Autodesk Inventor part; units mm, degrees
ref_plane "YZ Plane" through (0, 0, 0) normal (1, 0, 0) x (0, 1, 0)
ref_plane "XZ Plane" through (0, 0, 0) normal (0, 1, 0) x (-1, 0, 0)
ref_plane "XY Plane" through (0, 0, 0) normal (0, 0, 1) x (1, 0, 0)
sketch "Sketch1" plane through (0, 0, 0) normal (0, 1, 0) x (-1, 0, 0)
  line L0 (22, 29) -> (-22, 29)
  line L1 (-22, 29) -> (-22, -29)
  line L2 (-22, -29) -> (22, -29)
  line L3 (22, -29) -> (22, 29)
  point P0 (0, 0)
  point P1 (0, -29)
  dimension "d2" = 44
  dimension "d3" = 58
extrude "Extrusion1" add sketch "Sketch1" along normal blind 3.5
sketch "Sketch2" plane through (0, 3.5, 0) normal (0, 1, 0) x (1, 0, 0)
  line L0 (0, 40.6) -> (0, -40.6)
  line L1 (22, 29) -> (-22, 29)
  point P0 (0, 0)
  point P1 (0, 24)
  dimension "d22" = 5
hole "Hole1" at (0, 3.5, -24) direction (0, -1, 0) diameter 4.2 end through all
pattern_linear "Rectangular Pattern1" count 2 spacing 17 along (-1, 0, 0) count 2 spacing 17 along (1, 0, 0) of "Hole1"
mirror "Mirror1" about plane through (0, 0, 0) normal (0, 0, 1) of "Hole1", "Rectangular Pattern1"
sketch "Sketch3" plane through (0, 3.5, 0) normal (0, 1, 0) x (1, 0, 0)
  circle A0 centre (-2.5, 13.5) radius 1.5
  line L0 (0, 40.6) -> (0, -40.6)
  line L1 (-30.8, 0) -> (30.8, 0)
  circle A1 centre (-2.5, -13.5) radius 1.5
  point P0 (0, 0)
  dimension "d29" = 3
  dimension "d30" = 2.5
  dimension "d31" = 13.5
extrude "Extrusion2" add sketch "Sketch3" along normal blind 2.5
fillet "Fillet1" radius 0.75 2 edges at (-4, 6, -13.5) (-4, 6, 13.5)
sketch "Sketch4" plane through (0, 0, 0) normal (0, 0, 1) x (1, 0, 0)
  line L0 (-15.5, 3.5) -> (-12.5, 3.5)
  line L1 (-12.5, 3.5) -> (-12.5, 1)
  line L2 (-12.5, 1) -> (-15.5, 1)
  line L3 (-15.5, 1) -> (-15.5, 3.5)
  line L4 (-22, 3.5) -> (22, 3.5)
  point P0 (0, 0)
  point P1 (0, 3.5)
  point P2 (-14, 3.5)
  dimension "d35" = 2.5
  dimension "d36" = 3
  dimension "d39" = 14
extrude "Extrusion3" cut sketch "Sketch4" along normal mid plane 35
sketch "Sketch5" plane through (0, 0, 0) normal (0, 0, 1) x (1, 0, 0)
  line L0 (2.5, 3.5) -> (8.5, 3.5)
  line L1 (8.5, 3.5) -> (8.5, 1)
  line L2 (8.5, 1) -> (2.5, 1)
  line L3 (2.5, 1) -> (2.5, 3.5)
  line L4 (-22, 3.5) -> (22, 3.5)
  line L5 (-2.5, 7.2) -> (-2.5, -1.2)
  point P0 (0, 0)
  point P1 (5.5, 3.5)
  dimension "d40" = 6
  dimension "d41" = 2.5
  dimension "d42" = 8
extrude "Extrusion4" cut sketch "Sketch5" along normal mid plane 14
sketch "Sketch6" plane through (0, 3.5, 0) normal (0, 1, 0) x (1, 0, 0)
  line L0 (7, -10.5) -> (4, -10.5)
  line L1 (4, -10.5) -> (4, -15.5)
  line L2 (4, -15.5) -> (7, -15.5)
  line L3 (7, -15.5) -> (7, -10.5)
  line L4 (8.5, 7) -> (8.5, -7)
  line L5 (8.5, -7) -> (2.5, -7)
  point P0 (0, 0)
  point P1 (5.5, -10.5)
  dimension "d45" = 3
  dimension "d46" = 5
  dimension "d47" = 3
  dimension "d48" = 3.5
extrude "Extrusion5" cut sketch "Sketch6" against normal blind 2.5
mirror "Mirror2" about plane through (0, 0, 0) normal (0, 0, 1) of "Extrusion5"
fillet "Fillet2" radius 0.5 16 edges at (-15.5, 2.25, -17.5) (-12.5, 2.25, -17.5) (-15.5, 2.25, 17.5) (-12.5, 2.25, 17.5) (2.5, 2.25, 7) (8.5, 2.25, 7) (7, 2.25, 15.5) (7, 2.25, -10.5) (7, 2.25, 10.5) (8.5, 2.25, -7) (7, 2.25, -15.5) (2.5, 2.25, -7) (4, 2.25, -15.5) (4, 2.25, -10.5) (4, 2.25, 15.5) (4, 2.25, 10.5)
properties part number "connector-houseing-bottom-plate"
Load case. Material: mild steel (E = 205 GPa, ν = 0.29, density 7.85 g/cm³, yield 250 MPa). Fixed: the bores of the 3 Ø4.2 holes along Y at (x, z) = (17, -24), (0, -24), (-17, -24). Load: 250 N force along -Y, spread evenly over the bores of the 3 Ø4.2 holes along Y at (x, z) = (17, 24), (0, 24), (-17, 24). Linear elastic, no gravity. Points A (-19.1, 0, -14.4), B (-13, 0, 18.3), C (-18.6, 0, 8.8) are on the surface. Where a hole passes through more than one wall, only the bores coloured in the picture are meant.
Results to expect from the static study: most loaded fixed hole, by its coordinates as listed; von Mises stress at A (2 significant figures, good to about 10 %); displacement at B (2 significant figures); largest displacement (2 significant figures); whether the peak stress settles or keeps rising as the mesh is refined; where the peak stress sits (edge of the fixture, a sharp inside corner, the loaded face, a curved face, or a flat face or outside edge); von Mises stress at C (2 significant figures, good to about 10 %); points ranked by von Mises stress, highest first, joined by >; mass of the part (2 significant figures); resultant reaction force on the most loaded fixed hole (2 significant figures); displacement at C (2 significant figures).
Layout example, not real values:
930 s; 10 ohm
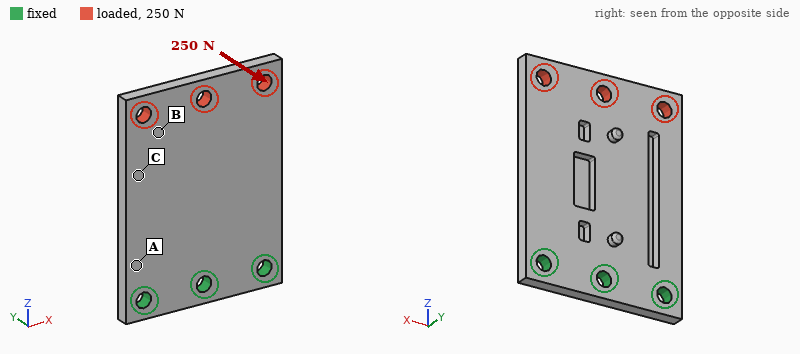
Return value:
(0, -24); 110 MPa; 0.24 mm; 0.33 mm; keeps rising; edge of the fixture; 44 MPa; A > C > B; 64 g; 170 N; 0.15 mm
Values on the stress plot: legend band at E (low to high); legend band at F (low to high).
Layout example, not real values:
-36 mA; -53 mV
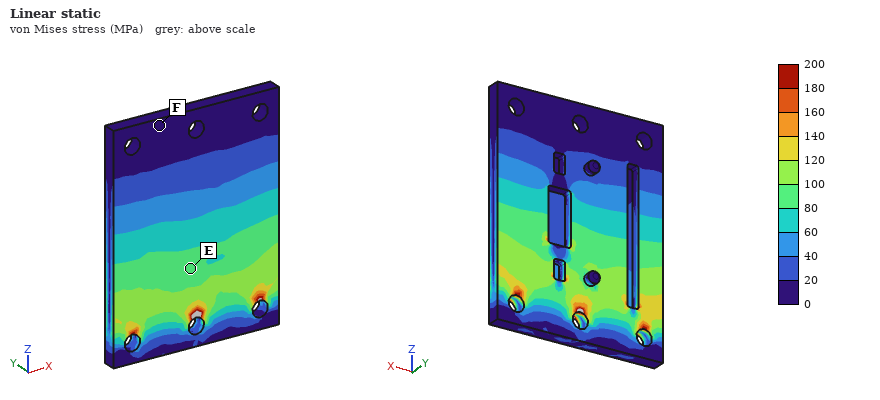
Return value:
80 to 100 MPa; 0 to 20 MPa
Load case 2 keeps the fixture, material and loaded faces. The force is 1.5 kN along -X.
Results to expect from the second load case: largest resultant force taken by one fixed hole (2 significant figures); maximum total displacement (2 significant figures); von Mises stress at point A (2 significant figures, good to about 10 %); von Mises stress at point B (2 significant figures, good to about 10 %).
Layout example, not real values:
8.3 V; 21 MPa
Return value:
2.1 kN; 29 µm; 55 MPa; 24 MPa
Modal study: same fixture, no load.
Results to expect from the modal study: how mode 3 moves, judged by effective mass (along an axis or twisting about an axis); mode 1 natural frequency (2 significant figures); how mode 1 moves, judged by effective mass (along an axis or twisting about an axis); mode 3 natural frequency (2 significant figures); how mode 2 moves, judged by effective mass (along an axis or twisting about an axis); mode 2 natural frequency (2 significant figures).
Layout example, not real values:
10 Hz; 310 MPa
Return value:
along Y; 1100 Hz; along Y; 6600 Hz; twisting about Z; 2800 Hz
